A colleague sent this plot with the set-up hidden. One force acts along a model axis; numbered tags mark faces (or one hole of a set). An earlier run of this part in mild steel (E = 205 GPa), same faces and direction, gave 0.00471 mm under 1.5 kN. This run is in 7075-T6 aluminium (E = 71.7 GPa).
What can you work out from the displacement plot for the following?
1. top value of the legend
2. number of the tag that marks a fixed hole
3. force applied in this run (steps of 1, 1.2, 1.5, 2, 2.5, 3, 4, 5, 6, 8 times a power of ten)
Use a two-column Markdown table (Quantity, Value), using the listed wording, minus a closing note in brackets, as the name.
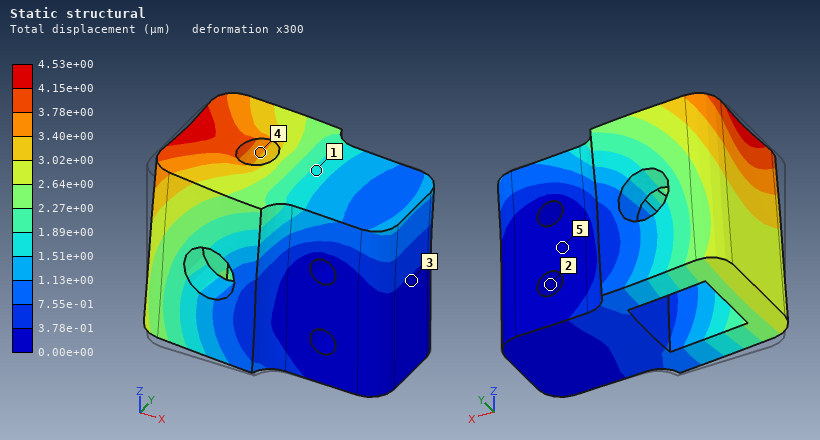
| Quantity | Value |
|---|---|
| top value of the legend | 4.53e+00 µm |
| number of the tag that marks a fixed hole | 2 |
| force applied in this run | 500 N |
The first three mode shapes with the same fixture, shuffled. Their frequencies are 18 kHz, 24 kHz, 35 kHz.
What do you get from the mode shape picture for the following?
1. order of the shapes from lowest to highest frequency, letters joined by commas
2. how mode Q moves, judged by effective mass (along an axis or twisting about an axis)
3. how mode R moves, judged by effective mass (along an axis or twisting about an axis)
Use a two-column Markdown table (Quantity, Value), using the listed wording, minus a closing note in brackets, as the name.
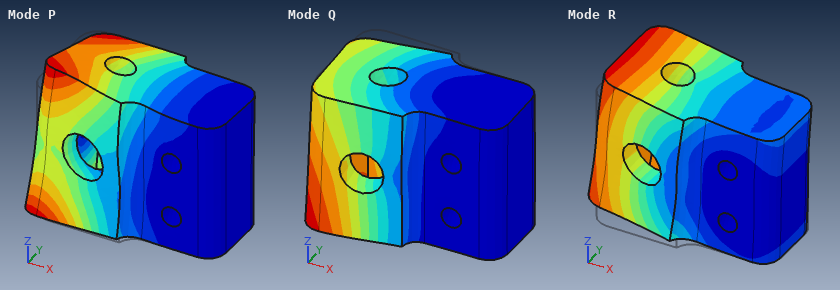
| Quantity | Value |
|---|---|
| order of the shapes from lowest to highest frequency, letters joined by commas | Q, R, P |
| how mode Q moves, judged by effective mass | along Y |
| how mode R moves, judged by effective mass | along Z |
